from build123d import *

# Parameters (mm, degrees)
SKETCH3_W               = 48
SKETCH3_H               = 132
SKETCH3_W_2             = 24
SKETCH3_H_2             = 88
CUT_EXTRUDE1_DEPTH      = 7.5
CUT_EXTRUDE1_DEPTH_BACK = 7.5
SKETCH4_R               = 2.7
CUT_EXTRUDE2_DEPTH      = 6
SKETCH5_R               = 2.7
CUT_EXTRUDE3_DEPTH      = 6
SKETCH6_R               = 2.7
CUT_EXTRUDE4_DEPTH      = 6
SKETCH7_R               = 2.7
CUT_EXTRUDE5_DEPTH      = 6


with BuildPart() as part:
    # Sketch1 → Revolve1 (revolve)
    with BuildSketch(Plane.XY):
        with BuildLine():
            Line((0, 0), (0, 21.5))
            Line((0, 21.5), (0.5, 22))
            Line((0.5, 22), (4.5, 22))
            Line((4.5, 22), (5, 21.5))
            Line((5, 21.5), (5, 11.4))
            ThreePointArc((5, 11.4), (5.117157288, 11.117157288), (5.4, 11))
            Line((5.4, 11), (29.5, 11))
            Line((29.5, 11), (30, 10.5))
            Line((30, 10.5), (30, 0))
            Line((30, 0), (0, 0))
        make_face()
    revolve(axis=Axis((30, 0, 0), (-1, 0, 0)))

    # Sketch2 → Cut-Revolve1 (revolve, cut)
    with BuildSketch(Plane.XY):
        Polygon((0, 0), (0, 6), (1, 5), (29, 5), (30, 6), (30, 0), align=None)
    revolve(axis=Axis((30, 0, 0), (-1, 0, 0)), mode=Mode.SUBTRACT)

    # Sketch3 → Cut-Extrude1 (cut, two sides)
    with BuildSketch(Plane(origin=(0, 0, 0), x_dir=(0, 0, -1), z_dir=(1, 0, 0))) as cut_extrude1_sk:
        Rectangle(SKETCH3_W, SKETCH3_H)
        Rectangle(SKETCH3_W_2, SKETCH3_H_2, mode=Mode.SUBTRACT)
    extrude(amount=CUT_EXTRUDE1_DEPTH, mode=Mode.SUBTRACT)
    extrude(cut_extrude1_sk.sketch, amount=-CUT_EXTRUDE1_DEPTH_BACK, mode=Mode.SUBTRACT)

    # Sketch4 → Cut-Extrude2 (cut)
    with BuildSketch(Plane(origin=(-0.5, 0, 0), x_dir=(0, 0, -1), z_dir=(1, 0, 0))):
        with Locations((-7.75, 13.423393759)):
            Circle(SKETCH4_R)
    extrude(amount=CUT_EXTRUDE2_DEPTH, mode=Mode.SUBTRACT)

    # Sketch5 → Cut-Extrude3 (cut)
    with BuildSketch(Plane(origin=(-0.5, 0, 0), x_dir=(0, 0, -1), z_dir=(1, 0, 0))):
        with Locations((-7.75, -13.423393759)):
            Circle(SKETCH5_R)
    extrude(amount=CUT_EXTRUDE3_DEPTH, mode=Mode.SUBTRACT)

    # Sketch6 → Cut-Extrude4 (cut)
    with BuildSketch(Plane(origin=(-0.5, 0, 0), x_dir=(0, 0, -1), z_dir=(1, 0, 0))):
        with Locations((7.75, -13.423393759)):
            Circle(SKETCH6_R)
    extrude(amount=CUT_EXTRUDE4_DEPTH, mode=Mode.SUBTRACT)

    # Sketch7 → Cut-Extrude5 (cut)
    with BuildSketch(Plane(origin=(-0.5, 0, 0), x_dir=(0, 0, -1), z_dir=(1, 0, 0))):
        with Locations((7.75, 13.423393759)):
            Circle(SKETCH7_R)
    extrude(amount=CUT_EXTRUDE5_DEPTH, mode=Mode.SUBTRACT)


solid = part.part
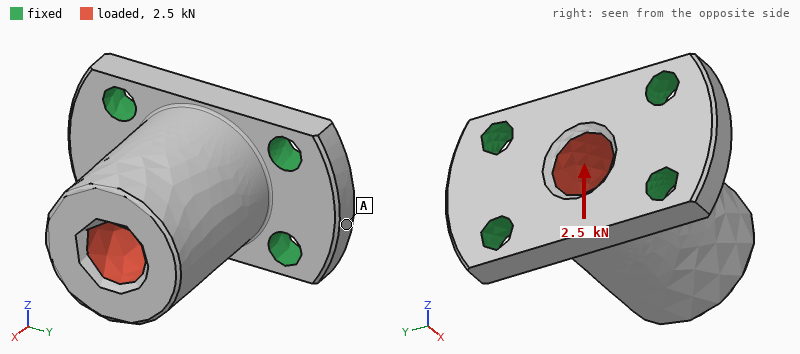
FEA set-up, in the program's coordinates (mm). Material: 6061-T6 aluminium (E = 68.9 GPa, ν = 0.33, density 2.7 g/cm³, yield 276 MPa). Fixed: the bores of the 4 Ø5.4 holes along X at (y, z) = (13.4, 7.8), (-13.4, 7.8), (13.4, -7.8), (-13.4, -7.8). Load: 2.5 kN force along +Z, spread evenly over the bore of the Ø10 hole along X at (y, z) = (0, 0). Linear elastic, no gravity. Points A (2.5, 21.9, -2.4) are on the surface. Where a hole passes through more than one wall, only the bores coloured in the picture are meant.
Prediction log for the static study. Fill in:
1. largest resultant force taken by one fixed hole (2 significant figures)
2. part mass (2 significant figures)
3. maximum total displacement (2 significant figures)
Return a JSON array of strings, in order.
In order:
["1.3 kN", "31 g", "37 µm"]
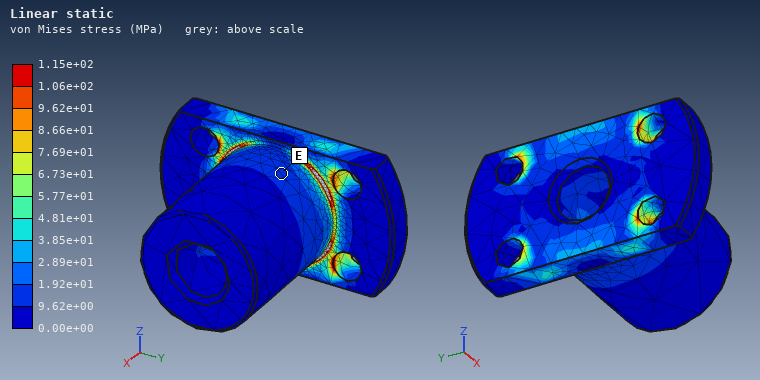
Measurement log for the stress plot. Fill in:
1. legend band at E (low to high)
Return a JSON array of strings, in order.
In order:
["9.62e+00 to 1.92e+01 MPa"]
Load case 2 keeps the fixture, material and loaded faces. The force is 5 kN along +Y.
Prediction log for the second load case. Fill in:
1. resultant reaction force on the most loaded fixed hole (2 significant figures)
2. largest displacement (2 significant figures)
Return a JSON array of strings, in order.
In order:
["1.9 kN", "38 µm"]
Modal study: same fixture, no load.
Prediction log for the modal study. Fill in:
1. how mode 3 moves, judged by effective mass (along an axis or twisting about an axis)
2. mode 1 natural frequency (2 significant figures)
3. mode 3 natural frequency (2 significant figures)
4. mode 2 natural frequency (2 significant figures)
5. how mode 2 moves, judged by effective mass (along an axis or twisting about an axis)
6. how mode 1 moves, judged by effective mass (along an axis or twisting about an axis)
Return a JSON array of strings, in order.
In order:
["along X", "9800 Hz", "25 kHz", "14 kHz", "along Y", "along Z"]
